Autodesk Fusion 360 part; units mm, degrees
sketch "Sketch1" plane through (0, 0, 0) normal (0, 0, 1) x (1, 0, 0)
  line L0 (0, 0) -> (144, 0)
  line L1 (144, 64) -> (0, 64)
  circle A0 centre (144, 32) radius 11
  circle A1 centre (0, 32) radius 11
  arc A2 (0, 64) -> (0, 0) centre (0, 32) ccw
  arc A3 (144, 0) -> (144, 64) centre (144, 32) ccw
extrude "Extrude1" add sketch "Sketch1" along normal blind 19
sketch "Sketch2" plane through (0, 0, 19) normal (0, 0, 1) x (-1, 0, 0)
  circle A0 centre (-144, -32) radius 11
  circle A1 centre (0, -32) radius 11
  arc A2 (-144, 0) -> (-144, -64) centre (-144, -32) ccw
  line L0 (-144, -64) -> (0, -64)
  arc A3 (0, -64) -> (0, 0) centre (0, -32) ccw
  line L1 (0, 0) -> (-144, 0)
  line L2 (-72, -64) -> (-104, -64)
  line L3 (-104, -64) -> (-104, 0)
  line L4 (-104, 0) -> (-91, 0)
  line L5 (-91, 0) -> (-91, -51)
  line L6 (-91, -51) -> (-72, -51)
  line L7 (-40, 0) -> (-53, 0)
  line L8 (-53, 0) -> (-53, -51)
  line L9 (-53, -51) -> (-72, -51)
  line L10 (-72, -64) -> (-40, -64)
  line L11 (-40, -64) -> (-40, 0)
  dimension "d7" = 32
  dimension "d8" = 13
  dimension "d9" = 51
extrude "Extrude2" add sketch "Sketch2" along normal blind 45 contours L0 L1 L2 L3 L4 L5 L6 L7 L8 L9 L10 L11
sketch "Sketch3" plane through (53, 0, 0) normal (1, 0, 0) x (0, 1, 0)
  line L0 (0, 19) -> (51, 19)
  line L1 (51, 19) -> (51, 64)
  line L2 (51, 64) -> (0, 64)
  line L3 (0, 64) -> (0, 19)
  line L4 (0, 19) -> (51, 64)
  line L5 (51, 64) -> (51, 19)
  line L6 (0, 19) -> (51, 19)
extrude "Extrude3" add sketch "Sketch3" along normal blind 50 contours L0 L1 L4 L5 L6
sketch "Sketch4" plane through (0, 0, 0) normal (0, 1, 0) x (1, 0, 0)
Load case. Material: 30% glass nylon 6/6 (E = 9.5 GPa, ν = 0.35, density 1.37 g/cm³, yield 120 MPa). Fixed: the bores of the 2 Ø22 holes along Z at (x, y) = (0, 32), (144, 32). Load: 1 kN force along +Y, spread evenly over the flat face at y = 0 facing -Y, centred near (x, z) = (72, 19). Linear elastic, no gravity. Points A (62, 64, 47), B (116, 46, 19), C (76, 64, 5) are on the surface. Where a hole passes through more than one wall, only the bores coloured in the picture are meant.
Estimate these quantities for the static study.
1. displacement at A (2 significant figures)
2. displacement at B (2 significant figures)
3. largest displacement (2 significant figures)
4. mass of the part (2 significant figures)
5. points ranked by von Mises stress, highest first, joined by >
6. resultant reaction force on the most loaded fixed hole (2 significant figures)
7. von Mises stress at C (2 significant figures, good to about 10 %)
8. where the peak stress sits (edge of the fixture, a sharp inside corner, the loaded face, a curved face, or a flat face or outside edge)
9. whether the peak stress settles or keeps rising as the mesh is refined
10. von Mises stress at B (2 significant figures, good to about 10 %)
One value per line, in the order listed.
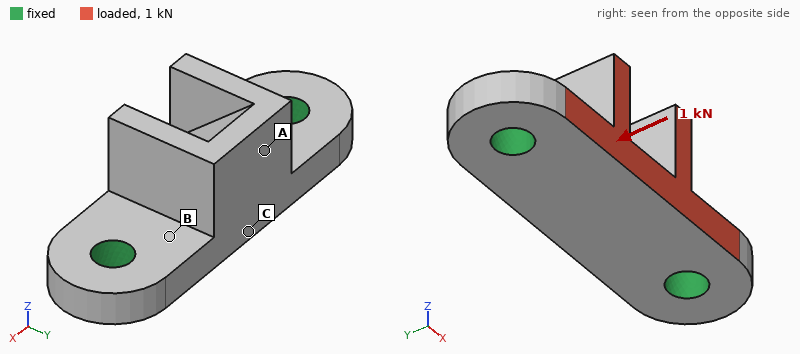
24 µm
6.7 µm
31 µm
500 g
B > C > A
500 N
0.75 MPa
edge of the fixture
keeps rising
1.4 MPa
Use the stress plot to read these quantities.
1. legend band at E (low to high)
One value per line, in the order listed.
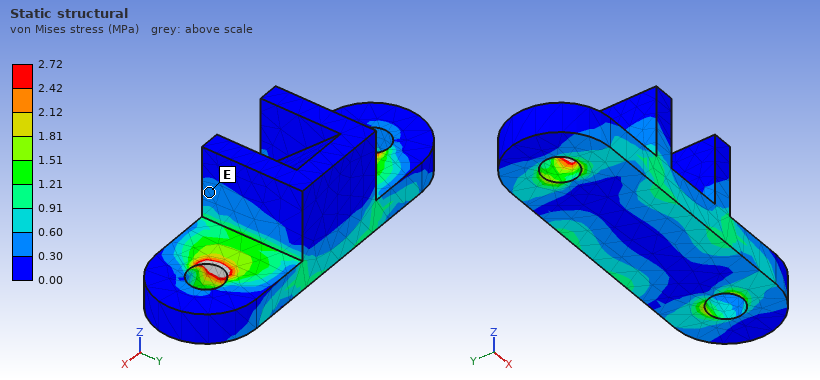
0.30 to 0.60 MPa
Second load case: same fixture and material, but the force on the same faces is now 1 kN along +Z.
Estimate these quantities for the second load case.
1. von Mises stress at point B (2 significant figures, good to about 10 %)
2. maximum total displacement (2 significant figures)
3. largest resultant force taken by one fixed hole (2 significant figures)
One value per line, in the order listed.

1.9 MPa
68 µm
520 N
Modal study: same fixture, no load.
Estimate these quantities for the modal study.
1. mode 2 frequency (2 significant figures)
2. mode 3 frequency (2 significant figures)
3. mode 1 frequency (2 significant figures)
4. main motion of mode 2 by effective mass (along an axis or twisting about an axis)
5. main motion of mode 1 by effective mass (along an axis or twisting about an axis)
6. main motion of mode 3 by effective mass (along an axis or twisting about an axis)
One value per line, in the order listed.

2100 Hz
3000 Hz
1400 Hz
along Z
along Y
along X
